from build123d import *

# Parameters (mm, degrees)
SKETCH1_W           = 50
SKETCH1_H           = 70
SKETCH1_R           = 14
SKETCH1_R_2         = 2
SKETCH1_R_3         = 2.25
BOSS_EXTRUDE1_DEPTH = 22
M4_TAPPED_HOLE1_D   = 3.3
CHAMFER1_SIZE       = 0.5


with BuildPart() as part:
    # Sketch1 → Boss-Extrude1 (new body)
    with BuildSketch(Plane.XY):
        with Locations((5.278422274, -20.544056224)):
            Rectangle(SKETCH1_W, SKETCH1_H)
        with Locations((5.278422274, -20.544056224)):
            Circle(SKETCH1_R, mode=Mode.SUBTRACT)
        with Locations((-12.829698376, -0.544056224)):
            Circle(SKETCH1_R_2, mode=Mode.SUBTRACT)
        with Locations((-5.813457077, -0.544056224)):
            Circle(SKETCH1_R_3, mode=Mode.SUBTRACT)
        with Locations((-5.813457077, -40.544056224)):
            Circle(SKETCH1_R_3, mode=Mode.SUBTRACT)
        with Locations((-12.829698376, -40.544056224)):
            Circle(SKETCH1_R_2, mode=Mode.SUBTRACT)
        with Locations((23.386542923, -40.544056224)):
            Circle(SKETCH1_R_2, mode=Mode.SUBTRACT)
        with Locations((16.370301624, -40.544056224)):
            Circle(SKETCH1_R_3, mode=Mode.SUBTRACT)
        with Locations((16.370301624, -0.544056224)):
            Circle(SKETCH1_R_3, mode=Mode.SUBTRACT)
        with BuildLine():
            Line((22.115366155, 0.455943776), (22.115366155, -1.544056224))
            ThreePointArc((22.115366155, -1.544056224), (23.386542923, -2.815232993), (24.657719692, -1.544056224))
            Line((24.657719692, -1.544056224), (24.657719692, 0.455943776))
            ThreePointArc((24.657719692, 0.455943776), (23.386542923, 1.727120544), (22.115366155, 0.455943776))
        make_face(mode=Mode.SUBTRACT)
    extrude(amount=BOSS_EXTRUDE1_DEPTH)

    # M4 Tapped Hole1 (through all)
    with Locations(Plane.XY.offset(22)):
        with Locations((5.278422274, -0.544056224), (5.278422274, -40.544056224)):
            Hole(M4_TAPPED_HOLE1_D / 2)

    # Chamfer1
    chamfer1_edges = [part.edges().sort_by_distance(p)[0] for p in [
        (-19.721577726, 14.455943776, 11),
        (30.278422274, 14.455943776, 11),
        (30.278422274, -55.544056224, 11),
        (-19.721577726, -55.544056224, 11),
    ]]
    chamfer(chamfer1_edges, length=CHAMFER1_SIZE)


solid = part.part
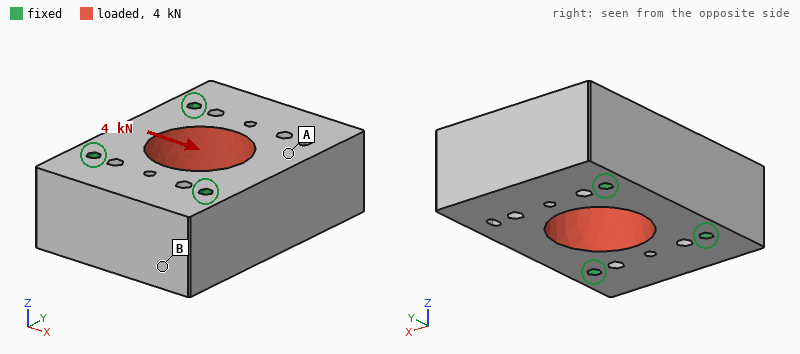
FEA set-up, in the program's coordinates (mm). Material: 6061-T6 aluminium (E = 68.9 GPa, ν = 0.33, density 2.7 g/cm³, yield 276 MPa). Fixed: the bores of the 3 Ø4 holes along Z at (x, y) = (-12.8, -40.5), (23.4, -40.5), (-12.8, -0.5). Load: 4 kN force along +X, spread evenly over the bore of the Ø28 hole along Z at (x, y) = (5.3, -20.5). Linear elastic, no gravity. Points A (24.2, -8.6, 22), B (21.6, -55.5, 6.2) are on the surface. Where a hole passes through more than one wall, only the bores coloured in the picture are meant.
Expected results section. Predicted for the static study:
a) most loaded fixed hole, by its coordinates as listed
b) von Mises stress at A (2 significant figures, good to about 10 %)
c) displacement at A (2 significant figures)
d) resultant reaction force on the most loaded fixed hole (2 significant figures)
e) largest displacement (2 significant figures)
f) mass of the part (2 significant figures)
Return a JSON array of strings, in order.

["(-12.8, -0.5)", "3.0 MPa", "2.7 µm", "1.9 kN", "3.2 µm", "160 g"]
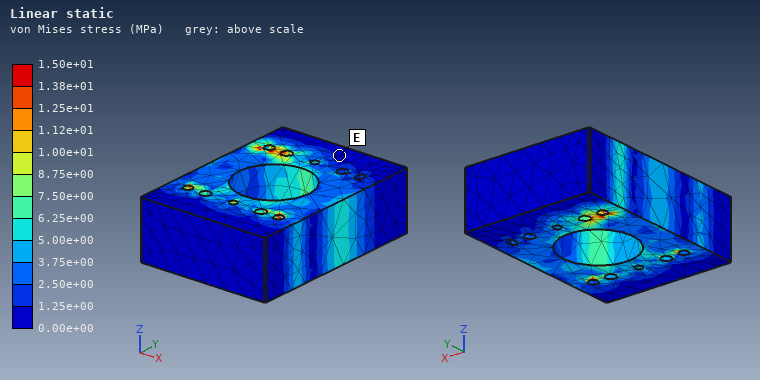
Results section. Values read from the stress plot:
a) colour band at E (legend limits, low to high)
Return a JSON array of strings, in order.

["0.00e+00 to 1.25e+00 MPa"]
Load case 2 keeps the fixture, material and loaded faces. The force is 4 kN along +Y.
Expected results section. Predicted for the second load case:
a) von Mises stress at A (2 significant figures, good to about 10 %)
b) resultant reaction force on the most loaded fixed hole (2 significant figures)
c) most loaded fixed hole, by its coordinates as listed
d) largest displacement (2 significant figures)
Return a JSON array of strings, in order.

["1.7 MPa", "1.8 kN", "(23.4, -40.5)", "2.4 µm"]
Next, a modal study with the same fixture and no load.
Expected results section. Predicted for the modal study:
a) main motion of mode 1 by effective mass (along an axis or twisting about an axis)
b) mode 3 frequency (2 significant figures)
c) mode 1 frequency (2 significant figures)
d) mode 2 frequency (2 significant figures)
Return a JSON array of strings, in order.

["along Z", "22 kHz", "8800 Hz", "17 kHz"]
